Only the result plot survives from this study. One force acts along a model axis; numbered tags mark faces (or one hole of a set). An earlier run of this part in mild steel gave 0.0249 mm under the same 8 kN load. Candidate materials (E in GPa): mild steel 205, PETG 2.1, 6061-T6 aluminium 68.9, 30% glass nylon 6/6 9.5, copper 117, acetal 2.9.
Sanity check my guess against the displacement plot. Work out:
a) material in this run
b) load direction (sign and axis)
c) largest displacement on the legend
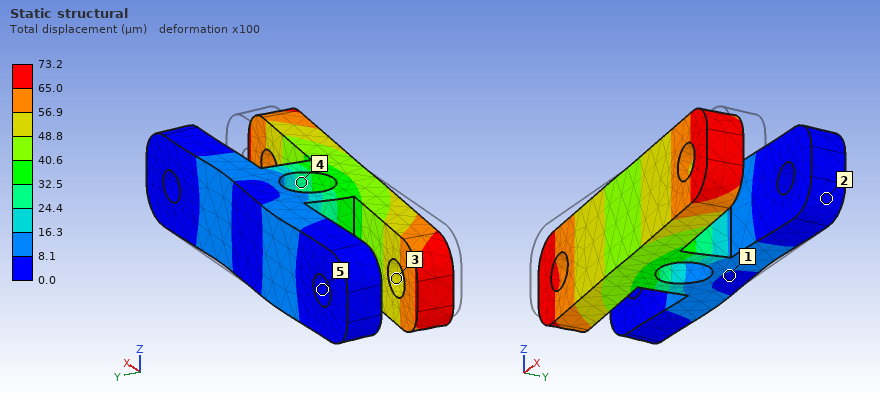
6061-T6 aluminium
-X
73.2 µm
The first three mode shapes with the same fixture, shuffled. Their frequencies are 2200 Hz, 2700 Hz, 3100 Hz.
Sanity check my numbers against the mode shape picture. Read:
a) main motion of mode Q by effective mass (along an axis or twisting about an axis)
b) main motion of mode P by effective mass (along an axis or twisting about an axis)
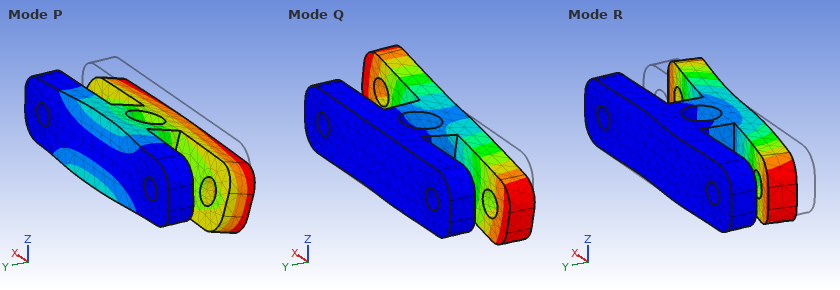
twisting about Y
along Z
